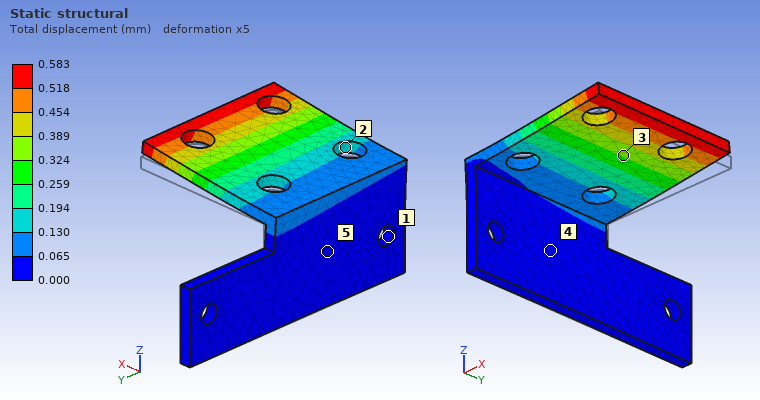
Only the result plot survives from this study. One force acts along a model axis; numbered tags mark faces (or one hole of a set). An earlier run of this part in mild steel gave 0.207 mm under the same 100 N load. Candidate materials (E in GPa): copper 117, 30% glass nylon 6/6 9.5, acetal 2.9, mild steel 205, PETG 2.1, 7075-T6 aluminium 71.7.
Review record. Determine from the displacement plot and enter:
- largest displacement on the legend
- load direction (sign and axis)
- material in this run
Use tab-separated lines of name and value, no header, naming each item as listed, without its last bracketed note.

largest displacement on the legend	0.583 mm
load direction	+Z
material in this run	7075-T6 aluminium
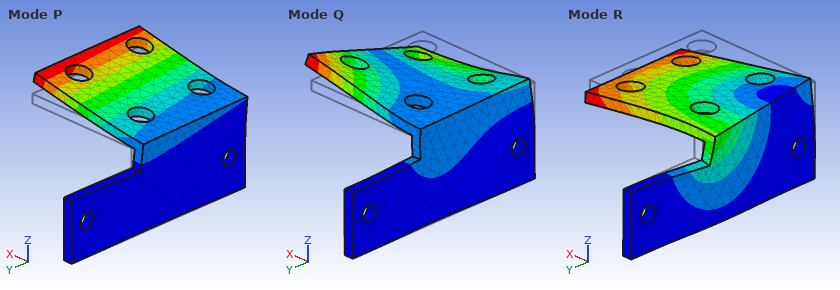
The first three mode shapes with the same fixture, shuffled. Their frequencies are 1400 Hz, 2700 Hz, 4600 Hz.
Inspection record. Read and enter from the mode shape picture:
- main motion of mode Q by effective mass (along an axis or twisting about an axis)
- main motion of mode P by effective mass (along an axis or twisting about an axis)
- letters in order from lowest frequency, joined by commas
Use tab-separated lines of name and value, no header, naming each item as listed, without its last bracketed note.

main motion of mode Q by effective mass	along X
main motion of mode P by effective mass	along Z
letters in order from lowest frequency, joined by commas	P, R, Q
